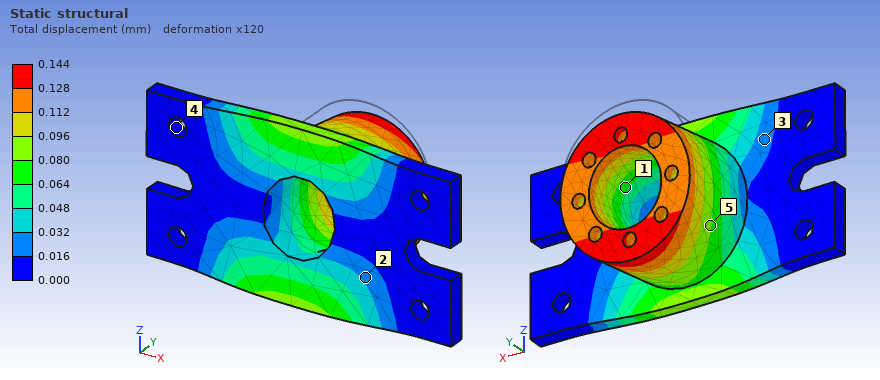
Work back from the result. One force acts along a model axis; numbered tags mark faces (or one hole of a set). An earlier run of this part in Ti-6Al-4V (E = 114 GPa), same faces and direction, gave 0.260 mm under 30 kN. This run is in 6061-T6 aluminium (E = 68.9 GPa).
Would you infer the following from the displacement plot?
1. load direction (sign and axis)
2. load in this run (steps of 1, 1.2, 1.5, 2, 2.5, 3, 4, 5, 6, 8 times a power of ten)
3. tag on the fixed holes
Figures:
-Z
10 kN
4
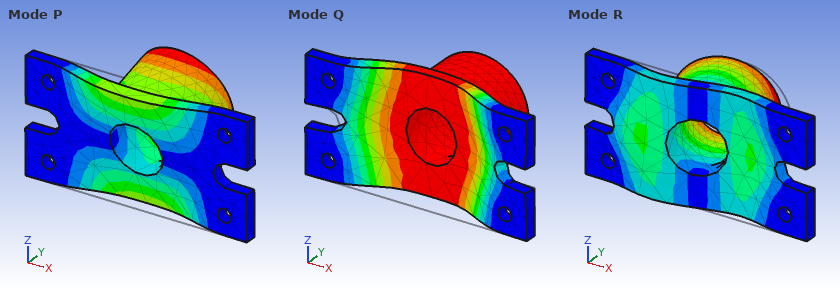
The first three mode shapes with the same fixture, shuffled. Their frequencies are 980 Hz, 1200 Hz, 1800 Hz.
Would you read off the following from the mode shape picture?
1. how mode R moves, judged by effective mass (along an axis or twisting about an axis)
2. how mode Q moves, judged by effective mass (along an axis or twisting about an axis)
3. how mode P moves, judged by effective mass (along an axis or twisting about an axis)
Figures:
along X
along Y
along Z
